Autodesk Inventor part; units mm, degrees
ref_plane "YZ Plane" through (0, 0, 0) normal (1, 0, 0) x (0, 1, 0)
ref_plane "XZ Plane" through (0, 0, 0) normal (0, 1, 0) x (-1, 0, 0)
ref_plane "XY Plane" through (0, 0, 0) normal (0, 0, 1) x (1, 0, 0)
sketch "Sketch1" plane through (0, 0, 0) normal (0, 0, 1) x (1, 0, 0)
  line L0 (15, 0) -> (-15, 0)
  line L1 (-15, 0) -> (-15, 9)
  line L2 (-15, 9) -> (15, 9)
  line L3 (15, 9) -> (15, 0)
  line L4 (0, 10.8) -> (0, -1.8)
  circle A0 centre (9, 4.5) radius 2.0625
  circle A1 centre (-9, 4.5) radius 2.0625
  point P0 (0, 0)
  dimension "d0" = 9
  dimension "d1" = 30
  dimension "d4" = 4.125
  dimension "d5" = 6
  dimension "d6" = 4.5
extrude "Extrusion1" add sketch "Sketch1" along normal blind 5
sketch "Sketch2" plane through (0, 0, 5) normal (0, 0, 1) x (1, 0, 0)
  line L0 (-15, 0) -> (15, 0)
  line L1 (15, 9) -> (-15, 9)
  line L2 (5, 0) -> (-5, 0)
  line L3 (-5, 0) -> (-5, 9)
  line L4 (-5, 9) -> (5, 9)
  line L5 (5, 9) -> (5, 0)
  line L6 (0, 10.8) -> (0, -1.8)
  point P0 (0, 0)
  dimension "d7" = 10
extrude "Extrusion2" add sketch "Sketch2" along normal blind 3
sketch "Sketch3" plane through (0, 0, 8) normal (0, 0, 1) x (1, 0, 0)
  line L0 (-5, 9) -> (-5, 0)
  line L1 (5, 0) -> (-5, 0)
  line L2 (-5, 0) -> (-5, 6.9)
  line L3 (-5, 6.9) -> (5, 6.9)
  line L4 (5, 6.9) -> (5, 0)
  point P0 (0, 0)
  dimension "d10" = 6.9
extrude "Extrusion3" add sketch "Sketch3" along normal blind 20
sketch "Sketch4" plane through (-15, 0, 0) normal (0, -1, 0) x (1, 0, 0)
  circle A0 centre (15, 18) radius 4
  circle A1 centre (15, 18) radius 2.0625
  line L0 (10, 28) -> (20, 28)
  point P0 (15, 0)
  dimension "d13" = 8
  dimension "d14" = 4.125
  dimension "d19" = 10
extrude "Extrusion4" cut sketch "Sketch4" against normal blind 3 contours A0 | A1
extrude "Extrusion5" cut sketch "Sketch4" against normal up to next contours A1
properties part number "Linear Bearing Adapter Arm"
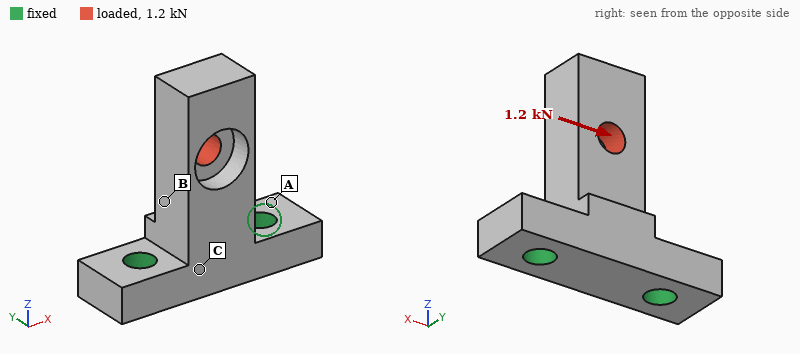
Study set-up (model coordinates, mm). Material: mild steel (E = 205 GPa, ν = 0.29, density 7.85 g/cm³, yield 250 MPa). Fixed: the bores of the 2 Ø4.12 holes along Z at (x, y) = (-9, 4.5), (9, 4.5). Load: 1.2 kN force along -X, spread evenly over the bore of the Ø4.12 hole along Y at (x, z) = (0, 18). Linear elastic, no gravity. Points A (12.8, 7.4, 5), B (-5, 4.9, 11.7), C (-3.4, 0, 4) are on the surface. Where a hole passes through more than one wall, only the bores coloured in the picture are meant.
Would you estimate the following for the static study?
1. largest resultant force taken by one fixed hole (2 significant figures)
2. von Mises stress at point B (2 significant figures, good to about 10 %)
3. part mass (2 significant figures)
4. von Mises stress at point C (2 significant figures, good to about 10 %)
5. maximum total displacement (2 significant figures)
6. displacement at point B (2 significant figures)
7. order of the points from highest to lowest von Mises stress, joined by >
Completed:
1.5 kN
85 MPa
21 g
42 MPa
35 µm
10 µm
B > C > A
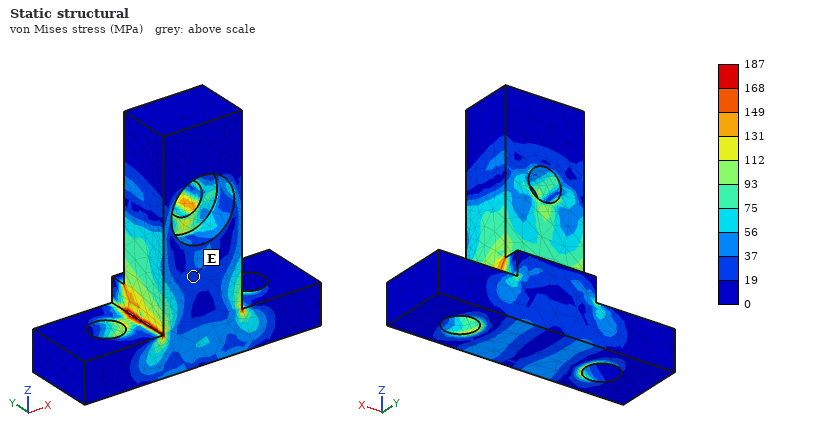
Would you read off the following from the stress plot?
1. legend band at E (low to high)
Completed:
19 to 37 MPa
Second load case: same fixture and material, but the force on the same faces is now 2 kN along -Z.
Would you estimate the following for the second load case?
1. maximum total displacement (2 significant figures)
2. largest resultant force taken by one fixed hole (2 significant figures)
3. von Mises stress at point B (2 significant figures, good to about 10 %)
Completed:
14 µm
1.0 kN
47 MPa
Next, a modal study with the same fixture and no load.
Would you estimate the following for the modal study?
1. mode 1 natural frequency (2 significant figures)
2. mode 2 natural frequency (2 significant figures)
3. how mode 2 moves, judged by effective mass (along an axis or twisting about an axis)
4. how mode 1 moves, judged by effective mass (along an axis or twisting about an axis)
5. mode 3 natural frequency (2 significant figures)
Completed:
7000 Hz
11 kHz
along X
along Y
25 kHz
